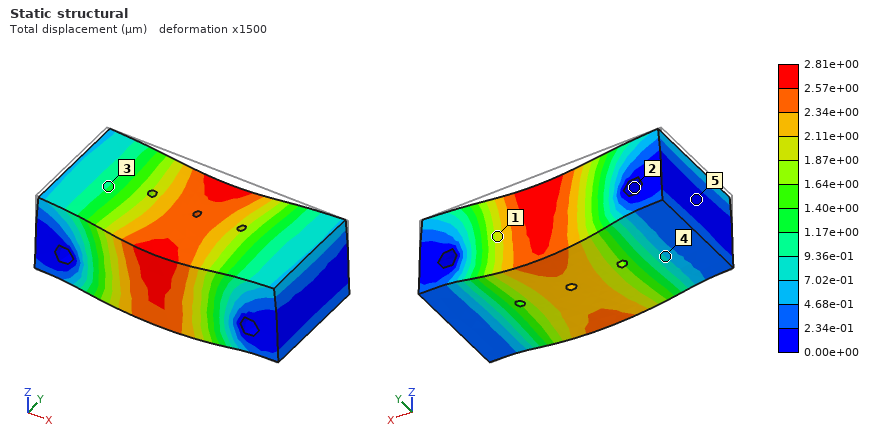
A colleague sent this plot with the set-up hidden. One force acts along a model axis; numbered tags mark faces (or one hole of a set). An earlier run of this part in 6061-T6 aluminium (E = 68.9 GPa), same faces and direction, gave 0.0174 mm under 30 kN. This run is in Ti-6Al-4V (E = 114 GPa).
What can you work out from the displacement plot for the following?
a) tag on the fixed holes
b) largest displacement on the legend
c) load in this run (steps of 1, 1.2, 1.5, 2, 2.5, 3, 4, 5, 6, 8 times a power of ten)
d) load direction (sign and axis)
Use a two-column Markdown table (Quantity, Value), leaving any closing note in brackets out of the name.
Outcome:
| Quantity | Value |
|---|---|
| tag on the fixed holes | 2 |
| largest displacement on the legend | 2.81e+00 µm |
| load in this run | 8 kN |
| load direction | -Z |
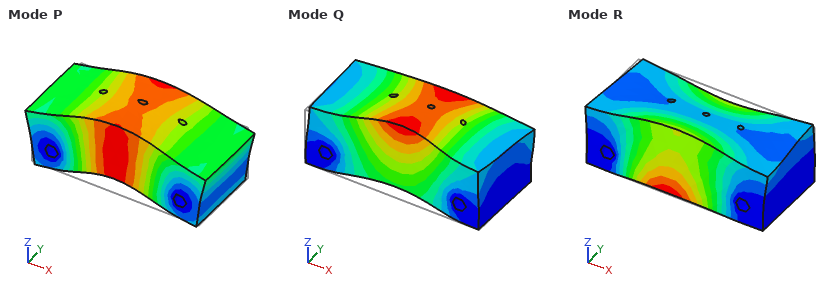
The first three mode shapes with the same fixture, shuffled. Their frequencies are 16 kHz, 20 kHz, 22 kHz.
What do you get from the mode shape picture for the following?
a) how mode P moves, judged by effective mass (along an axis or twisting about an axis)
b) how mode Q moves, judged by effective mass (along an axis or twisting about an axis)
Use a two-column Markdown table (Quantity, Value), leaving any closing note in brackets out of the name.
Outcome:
| Quantity | Value |
|---|---|
| how mode P moves, judged by effective mass | along Z |
| how mode Q moves, judged by effective mass | along Y |
